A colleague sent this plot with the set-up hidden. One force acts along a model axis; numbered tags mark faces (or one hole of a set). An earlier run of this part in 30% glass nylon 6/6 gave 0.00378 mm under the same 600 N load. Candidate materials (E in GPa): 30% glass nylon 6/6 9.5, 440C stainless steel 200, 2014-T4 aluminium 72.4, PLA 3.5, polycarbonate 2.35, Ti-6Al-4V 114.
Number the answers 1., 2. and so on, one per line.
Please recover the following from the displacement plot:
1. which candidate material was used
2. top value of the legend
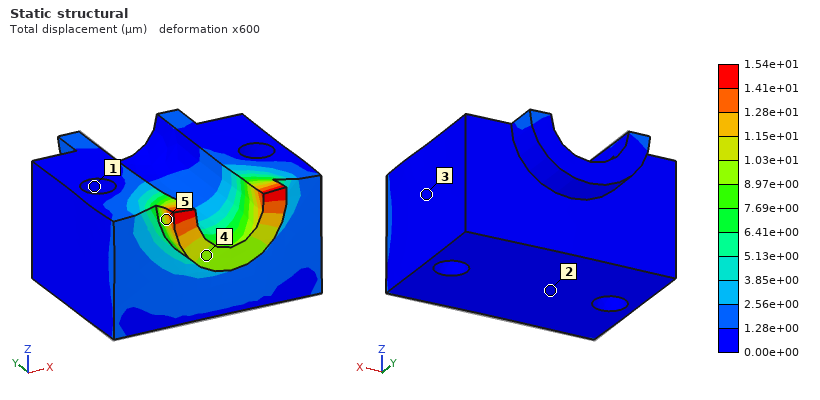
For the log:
1. polycarbonate
2. 1.54e+01 µm
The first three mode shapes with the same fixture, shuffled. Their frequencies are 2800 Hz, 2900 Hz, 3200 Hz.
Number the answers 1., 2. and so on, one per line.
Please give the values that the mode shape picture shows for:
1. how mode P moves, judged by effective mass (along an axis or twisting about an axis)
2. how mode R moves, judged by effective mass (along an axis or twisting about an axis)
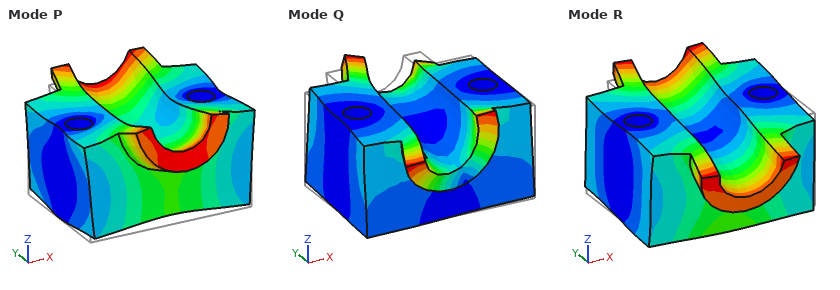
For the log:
1. along Z
2. twisting about X
